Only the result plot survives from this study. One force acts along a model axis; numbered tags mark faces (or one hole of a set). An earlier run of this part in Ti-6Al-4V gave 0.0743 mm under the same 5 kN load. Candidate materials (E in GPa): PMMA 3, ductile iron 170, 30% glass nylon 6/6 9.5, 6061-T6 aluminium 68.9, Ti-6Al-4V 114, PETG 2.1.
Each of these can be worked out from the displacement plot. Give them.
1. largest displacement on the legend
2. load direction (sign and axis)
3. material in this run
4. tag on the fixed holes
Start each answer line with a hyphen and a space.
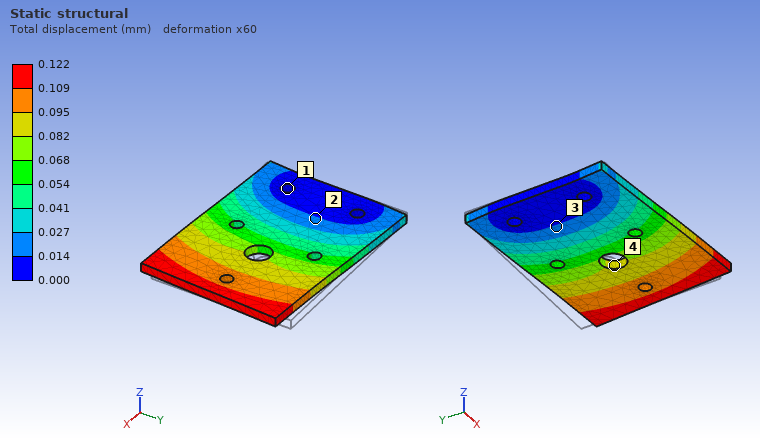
- 0.122 mm
- -Y
- 6061-T6 aluminium
- 1
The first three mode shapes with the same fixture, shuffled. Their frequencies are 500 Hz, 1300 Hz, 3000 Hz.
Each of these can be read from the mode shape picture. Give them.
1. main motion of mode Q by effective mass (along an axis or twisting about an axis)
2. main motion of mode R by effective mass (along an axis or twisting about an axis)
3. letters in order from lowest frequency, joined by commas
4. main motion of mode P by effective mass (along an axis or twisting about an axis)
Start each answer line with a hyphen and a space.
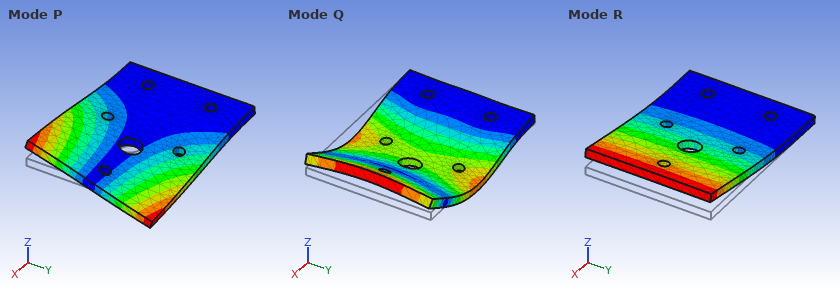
- along Z
- along Z
- R, P, Q
- twisting about X
